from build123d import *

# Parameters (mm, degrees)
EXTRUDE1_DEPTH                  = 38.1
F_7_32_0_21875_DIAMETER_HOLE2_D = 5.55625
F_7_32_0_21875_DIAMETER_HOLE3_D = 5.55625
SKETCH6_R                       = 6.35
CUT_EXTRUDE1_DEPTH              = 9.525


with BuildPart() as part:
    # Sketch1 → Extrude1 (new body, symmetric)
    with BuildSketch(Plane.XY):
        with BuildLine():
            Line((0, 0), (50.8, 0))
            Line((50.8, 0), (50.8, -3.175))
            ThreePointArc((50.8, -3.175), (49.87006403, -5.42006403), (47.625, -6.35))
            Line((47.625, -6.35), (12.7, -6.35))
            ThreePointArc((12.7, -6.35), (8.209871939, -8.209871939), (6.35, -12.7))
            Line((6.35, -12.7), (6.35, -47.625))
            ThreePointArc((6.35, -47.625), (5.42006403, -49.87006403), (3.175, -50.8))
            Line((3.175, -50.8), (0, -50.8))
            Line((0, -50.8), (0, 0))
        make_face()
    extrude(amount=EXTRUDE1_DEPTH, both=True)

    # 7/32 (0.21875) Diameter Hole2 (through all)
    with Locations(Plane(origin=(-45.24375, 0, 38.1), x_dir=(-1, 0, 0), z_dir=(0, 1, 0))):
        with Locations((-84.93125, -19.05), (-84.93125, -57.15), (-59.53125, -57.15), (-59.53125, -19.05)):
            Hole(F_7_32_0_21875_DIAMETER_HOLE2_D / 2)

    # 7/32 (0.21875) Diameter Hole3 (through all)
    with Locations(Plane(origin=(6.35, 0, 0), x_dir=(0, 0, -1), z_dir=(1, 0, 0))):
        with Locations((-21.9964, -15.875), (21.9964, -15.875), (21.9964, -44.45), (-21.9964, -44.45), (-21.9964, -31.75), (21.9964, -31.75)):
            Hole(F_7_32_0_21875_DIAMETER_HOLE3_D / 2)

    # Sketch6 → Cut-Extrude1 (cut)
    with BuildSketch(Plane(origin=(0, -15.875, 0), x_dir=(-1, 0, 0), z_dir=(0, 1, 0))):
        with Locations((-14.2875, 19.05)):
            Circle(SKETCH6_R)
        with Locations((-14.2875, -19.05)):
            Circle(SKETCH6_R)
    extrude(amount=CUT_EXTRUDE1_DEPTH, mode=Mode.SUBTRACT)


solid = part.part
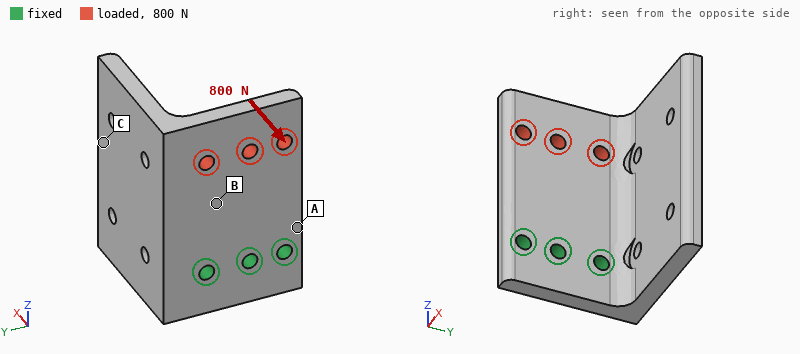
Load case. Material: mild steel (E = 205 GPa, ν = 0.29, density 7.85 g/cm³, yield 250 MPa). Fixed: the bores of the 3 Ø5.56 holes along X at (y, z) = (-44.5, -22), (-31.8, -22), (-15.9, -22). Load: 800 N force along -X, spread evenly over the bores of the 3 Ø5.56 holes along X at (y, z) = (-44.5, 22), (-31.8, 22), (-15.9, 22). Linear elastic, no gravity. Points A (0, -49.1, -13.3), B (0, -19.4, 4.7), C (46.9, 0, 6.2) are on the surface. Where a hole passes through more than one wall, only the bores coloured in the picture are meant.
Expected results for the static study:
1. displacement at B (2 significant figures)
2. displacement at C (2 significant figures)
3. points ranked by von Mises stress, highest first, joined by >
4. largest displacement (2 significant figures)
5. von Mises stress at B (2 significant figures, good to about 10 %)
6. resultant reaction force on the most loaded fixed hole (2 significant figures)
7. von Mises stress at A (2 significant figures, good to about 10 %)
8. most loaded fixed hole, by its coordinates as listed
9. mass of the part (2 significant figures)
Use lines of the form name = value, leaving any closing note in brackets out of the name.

displacement at B = 25 µm
displacement at C = 46 µm
points ranked by von Mises stress, highest first, joined by > = A > B > C
largest displacement = 91 µm
von Mises stress at B = 23 MPa
resultant reaction force on the most loaded fixed hole = 330 N
von Mises stress at A = 55 MPa
most loaded fixed hole, by its coordinates as listed = (-31.8, -22)
mass of the part = 350 g
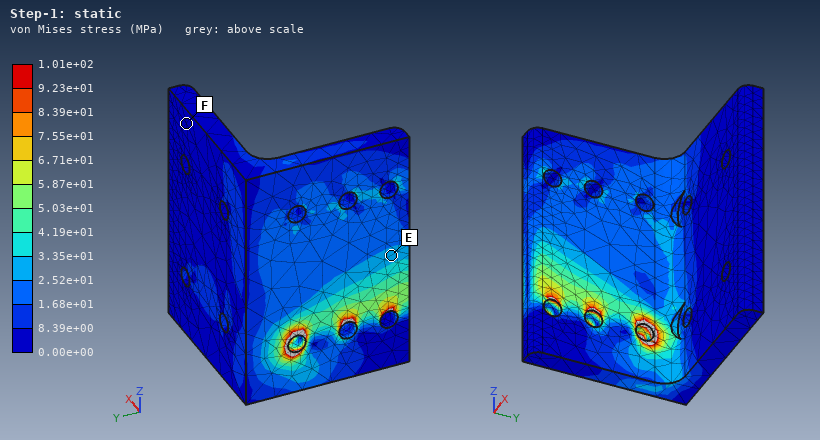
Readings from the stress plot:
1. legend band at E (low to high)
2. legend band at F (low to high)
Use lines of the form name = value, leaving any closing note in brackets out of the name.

legend band at E = 2.52e+01 to 3.35e+01 MPa
legend band at F = 0.00e+00 to 8.39e+00 MPa
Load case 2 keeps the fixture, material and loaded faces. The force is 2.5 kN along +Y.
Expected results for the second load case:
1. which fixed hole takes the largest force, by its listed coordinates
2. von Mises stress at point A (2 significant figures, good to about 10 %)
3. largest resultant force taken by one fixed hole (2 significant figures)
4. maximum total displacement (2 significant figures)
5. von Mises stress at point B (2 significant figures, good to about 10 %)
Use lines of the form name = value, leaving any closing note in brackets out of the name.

which fixed hole takes the largest force, by its listed coordinates = (-15.9, -22)
von Mises stress at point A = 32 MPa
largest resultant force taken by one fixed hole = 3.8 kN
maximum total displacement = 17 µm
von Mises stress at point B = 19 MPa
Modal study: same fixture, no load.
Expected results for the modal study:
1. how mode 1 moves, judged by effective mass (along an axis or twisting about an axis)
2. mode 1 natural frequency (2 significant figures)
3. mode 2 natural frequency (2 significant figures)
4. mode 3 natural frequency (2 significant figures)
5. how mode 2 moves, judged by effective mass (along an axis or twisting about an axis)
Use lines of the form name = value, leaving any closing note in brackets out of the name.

how mode 1 moves, judged by effective mass = along X
mode 1 natural frequency = 1200 Hz
mode 2 natural frequency = 1600 Hz
mode 3 natural frequency = 3300 Hz
how mode 2 moves, judged by effective mass = along Y
